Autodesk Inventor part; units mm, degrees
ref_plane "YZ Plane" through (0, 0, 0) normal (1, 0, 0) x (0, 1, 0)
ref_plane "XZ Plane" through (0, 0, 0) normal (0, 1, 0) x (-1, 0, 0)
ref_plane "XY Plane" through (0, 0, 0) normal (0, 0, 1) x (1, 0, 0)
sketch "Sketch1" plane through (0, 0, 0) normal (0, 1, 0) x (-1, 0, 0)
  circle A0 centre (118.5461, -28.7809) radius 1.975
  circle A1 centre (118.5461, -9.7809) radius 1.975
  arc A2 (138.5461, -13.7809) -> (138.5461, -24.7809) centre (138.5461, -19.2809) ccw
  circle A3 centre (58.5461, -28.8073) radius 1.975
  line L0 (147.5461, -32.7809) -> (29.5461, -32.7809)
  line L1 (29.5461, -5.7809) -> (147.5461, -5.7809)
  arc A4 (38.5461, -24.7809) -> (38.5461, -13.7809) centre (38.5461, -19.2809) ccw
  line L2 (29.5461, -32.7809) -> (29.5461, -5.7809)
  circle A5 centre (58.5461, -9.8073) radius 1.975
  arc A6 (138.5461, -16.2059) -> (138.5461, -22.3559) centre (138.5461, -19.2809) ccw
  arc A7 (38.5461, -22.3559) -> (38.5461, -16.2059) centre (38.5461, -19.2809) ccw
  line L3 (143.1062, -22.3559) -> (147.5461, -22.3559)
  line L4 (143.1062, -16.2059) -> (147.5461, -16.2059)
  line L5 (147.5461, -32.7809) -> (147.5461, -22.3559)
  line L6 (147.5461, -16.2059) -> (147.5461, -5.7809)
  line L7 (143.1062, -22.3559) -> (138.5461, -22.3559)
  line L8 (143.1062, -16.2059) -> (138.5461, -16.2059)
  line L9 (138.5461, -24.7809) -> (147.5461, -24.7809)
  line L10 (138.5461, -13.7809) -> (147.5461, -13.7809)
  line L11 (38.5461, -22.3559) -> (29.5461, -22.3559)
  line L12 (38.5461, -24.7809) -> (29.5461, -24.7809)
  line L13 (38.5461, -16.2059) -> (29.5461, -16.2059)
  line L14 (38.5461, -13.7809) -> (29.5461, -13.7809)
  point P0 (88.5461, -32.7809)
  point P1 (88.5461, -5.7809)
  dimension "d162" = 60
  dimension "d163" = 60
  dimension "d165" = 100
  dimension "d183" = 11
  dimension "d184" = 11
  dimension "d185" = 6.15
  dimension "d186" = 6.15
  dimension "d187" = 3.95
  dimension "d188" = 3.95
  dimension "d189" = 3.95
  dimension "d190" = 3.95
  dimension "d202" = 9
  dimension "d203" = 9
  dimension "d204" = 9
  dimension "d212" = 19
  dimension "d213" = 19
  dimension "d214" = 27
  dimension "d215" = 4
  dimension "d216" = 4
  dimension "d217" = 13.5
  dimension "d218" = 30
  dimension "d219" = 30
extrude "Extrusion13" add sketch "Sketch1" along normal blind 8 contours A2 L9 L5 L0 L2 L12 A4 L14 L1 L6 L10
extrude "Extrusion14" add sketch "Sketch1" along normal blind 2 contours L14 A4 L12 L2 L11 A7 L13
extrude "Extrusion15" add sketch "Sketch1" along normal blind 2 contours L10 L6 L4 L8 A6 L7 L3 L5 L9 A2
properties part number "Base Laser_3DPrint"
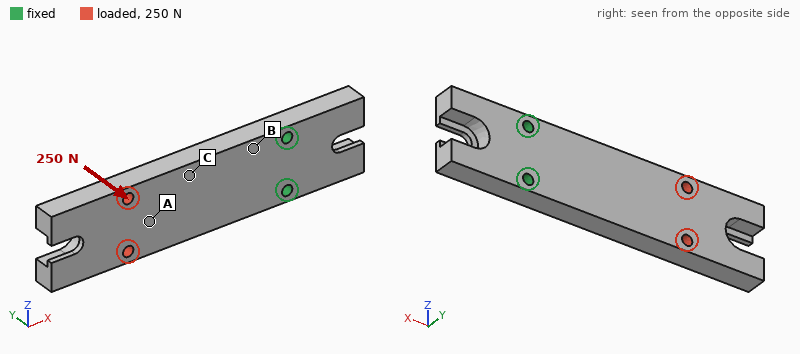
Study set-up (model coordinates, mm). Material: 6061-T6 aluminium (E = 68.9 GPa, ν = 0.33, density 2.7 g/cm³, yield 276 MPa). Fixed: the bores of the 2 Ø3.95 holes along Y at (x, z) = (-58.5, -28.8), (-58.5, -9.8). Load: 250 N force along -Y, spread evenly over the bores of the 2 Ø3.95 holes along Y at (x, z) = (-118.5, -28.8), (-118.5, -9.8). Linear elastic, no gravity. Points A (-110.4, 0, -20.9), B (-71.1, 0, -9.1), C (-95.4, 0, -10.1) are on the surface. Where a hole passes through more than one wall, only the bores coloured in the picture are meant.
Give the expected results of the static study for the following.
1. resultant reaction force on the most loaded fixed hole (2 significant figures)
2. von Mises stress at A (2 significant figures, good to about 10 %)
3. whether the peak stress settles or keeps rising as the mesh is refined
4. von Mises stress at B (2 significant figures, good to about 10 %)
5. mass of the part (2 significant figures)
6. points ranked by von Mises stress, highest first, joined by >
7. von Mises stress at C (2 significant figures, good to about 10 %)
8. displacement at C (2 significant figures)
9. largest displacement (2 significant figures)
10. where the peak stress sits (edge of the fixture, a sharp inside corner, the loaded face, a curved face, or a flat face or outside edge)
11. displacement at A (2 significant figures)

130 N
7.2 MPa
keeps rising
42 MPa
62 g
B > C > A
20 MPa
0.11 mm
0.40 mm
edge of the fixture
0.19 mm
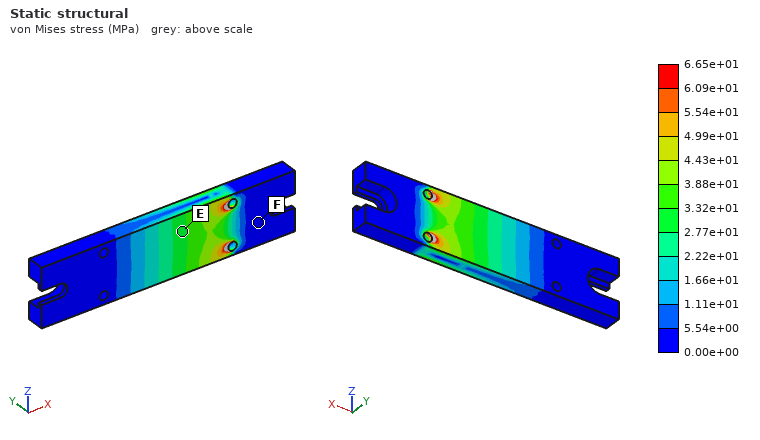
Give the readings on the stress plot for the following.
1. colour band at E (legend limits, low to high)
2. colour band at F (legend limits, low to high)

2.77e+01 to 3.32e+01 MPa
0.00e+00 to 5.54e+00 MPa
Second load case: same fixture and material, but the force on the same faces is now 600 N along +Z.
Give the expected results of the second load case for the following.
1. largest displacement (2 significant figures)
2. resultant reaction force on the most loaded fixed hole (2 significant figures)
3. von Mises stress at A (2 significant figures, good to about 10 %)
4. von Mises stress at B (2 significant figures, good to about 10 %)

90 µm
1.8 kN
7.0 MPa
22 MPa
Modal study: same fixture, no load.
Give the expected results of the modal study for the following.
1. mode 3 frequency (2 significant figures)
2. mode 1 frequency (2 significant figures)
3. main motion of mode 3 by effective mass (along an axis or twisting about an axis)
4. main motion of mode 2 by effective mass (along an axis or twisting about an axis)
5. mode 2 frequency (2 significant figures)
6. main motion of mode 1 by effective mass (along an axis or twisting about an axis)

4800 Hz
900 Hz
twisting about X
along Z
2900 Hz
along Y
